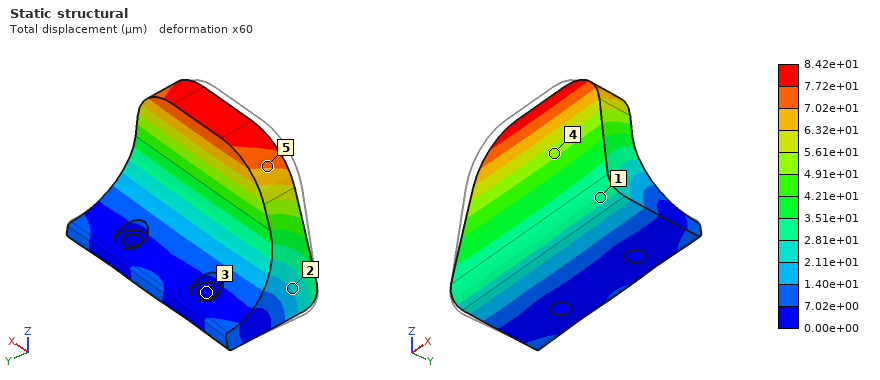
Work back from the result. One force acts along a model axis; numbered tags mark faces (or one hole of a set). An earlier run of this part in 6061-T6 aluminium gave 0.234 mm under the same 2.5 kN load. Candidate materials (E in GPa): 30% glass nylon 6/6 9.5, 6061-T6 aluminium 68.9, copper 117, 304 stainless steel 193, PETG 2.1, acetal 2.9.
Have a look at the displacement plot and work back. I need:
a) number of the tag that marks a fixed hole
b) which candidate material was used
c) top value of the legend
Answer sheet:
3
304 stainless steel
8.42e+01 µm
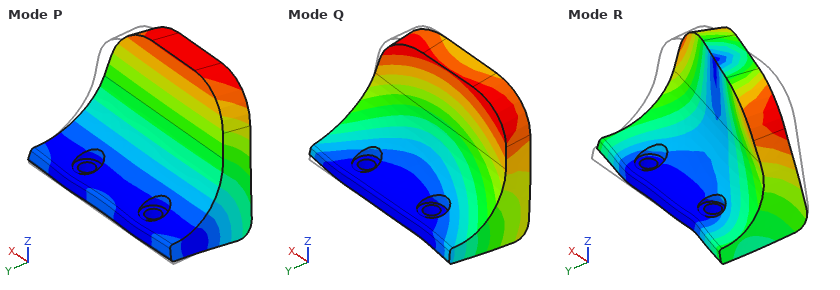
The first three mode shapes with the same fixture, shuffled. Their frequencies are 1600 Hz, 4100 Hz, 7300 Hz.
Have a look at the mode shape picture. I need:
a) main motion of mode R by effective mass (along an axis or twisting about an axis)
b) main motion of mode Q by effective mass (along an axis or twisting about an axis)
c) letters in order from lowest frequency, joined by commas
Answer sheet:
along X
along X
P, Q, R
